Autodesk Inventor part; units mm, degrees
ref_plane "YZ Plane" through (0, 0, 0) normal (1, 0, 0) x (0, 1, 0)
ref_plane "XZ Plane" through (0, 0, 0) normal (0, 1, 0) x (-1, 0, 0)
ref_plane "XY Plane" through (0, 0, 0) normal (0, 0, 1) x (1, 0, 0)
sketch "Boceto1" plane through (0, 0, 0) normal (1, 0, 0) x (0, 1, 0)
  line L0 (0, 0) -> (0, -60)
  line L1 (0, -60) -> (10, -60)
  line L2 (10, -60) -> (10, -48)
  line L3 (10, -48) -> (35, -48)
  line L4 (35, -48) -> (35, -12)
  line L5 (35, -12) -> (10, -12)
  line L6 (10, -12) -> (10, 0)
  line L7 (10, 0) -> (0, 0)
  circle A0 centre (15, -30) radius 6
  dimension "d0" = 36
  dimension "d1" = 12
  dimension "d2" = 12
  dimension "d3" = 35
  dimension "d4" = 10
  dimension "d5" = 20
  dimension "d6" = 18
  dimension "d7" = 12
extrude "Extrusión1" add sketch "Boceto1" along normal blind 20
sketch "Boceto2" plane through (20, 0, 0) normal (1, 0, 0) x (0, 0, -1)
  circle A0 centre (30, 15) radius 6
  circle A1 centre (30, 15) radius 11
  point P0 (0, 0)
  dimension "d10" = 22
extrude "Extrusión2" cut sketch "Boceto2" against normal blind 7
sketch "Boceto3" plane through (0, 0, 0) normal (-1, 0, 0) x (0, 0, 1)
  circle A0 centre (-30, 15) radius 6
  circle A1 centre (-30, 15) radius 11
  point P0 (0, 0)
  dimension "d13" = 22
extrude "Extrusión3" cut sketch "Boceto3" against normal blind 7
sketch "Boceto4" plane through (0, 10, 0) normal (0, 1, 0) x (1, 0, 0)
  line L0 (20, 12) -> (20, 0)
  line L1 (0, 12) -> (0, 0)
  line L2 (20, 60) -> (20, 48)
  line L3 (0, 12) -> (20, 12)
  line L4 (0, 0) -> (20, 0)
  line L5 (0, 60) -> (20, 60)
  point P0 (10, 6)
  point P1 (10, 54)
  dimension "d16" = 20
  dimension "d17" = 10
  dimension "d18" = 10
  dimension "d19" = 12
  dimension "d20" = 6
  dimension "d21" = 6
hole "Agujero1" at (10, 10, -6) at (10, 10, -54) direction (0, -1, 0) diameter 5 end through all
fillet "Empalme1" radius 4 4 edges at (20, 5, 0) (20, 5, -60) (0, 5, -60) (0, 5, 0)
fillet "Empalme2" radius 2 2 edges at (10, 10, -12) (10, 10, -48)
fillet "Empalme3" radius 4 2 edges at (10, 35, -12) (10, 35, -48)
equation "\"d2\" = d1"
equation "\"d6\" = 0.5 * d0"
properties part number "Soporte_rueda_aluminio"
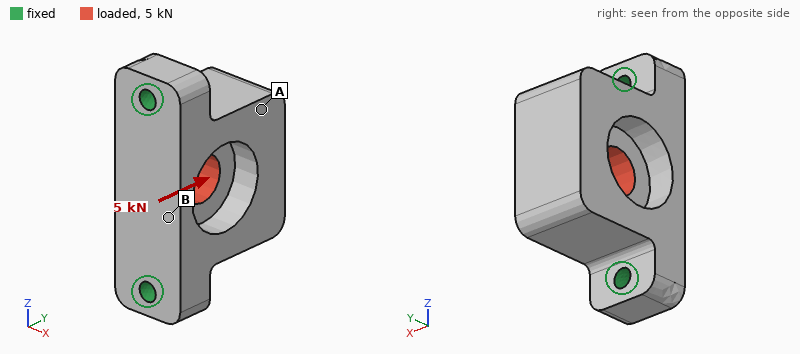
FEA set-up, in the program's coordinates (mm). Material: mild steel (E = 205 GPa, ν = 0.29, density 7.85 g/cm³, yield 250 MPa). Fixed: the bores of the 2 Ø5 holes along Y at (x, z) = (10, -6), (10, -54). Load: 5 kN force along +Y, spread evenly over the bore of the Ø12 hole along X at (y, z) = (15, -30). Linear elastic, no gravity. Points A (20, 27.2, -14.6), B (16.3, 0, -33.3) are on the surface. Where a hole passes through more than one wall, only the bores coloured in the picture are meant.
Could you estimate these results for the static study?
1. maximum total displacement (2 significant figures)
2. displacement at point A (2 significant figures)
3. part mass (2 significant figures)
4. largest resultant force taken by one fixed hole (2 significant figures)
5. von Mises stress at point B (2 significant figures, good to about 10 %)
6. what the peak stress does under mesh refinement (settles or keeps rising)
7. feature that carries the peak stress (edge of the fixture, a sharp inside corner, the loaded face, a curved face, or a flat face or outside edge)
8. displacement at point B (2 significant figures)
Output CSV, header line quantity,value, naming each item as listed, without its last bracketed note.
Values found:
quantity,value
maximum total displacement,5.8 µm
displacement at point A,3.4 µm
part mass,180 g
largest resultant force taken by one fixed hole,2.6 kN
von Mises stress at point B,21 MPa
what the peak stress does under mesh refinement,keeps rising
feature that carries the peak stress,edge of the fixture
displacement at point B,4.8 µm
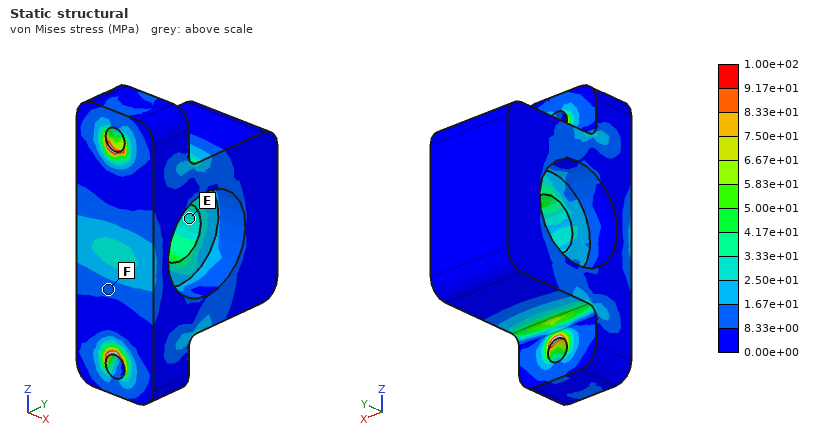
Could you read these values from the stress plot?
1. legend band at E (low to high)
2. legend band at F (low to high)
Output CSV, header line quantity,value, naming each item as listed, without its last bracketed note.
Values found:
quantity,value
legend band at E,2.50e+01 to 3.33e+01 MPa
legend band at F,8.33e+00 to 1.67e+01 MPa
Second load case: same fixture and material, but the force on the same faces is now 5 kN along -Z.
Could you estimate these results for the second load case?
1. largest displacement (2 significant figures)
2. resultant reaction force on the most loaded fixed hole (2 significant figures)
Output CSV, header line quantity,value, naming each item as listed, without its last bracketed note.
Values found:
quantity,value
largest displacement,4.5 µm
resultant reaction force on the most loaded fixed hole,2.7 kN
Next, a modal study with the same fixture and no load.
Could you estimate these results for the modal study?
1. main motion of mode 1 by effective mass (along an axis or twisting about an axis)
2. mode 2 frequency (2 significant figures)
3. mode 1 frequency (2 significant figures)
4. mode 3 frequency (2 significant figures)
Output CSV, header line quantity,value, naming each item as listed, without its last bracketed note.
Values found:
quantity,value
main motion of mode 1 by effective mass,along X
mode 2 frequency,13 kHz
mode 1 frequency,5900 Hz
mode 3 frequency,14 kHz
